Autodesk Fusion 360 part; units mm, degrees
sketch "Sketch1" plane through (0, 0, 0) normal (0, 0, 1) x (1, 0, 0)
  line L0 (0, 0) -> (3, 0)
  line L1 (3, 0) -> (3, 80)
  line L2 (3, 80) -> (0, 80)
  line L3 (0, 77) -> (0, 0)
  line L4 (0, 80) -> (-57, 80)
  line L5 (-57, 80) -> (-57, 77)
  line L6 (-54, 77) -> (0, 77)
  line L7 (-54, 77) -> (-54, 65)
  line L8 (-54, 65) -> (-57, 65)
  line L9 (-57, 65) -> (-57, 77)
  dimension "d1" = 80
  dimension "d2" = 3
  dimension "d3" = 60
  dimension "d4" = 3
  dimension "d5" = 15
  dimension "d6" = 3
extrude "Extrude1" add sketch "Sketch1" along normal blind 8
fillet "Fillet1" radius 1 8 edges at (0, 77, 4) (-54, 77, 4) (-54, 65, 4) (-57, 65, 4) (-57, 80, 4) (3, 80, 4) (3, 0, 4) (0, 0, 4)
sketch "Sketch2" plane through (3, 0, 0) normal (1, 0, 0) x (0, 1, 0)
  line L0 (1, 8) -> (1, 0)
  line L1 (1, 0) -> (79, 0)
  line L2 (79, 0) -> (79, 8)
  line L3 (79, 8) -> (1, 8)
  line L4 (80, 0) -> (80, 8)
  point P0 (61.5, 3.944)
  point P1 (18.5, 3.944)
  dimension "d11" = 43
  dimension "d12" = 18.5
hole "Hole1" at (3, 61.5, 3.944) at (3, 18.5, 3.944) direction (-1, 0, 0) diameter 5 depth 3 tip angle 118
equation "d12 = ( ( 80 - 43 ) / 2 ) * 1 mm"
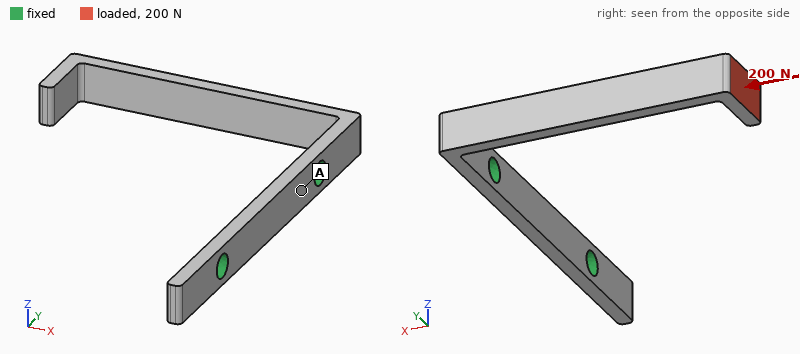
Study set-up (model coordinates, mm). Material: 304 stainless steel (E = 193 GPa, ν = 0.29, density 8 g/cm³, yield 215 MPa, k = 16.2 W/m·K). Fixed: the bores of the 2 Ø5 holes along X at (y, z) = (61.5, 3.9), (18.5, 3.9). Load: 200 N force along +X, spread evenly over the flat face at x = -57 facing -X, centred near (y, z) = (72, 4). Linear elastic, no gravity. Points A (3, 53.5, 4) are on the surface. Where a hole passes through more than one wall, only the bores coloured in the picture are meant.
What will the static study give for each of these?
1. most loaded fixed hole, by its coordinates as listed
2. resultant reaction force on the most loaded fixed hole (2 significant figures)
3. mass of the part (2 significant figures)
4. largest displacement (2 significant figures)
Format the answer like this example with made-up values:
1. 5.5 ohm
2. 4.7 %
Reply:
1. (61.5, 3.9)
2. 200 N
3. 28 g
4. 0.55 mm
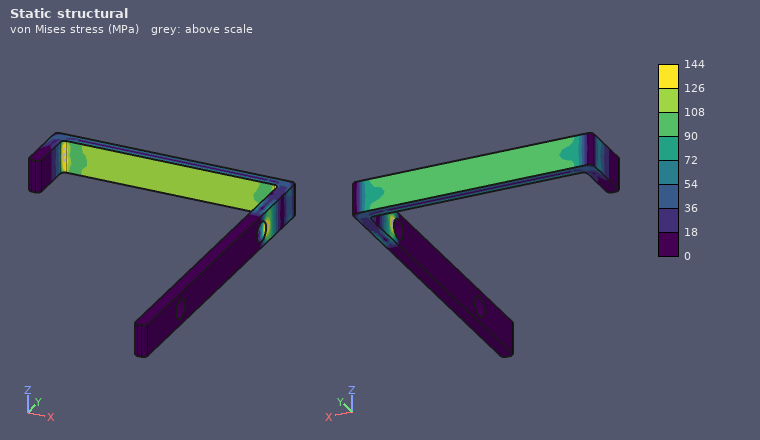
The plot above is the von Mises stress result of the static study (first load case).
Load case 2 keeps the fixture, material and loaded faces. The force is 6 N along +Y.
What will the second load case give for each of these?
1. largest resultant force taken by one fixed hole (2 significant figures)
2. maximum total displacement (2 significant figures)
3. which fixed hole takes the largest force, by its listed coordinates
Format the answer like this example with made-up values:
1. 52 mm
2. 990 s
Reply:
1. 6.0 N
2. 0.20 mm
3. (61.5, 3.9)
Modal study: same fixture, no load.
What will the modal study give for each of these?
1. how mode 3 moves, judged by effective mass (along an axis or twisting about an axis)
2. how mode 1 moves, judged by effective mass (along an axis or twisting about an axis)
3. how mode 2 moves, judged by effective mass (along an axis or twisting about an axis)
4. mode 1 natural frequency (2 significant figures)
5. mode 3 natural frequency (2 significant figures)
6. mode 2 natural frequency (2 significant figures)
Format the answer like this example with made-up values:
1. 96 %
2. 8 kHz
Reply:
1. along X
2. along Y
3. along Z
4. 390 Hz
5. 2200 Hz
6. 580 Hz
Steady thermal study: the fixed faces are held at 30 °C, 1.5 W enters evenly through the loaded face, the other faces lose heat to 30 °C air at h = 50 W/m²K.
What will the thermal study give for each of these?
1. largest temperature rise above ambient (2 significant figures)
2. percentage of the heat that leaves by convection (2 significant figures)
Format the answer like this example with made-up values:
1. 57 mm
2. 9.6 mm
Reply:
1. 57 K
2. 97 %
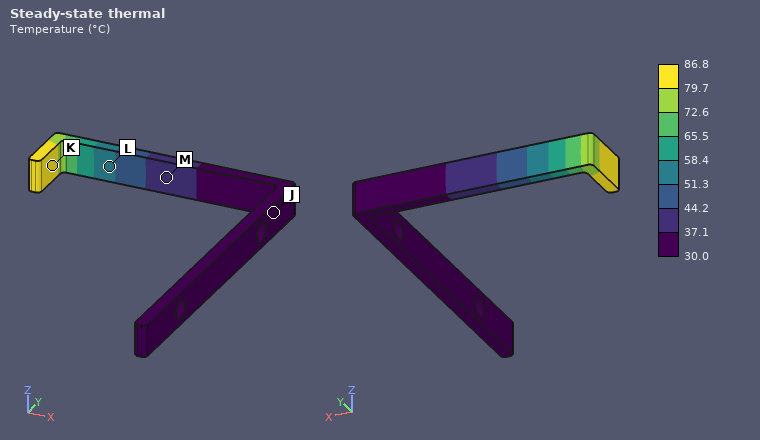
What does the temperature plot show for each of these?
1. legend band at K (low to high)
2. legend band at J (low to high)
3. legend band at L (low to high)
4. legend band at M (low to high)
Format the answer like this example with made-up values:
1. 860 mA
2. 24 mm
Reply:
1. 79.7 to 86.8 °C
2. 30.0 to 37.1 °C
3. 51.3 to 58.4 °C
4. 37.1 to 44.2 °C
